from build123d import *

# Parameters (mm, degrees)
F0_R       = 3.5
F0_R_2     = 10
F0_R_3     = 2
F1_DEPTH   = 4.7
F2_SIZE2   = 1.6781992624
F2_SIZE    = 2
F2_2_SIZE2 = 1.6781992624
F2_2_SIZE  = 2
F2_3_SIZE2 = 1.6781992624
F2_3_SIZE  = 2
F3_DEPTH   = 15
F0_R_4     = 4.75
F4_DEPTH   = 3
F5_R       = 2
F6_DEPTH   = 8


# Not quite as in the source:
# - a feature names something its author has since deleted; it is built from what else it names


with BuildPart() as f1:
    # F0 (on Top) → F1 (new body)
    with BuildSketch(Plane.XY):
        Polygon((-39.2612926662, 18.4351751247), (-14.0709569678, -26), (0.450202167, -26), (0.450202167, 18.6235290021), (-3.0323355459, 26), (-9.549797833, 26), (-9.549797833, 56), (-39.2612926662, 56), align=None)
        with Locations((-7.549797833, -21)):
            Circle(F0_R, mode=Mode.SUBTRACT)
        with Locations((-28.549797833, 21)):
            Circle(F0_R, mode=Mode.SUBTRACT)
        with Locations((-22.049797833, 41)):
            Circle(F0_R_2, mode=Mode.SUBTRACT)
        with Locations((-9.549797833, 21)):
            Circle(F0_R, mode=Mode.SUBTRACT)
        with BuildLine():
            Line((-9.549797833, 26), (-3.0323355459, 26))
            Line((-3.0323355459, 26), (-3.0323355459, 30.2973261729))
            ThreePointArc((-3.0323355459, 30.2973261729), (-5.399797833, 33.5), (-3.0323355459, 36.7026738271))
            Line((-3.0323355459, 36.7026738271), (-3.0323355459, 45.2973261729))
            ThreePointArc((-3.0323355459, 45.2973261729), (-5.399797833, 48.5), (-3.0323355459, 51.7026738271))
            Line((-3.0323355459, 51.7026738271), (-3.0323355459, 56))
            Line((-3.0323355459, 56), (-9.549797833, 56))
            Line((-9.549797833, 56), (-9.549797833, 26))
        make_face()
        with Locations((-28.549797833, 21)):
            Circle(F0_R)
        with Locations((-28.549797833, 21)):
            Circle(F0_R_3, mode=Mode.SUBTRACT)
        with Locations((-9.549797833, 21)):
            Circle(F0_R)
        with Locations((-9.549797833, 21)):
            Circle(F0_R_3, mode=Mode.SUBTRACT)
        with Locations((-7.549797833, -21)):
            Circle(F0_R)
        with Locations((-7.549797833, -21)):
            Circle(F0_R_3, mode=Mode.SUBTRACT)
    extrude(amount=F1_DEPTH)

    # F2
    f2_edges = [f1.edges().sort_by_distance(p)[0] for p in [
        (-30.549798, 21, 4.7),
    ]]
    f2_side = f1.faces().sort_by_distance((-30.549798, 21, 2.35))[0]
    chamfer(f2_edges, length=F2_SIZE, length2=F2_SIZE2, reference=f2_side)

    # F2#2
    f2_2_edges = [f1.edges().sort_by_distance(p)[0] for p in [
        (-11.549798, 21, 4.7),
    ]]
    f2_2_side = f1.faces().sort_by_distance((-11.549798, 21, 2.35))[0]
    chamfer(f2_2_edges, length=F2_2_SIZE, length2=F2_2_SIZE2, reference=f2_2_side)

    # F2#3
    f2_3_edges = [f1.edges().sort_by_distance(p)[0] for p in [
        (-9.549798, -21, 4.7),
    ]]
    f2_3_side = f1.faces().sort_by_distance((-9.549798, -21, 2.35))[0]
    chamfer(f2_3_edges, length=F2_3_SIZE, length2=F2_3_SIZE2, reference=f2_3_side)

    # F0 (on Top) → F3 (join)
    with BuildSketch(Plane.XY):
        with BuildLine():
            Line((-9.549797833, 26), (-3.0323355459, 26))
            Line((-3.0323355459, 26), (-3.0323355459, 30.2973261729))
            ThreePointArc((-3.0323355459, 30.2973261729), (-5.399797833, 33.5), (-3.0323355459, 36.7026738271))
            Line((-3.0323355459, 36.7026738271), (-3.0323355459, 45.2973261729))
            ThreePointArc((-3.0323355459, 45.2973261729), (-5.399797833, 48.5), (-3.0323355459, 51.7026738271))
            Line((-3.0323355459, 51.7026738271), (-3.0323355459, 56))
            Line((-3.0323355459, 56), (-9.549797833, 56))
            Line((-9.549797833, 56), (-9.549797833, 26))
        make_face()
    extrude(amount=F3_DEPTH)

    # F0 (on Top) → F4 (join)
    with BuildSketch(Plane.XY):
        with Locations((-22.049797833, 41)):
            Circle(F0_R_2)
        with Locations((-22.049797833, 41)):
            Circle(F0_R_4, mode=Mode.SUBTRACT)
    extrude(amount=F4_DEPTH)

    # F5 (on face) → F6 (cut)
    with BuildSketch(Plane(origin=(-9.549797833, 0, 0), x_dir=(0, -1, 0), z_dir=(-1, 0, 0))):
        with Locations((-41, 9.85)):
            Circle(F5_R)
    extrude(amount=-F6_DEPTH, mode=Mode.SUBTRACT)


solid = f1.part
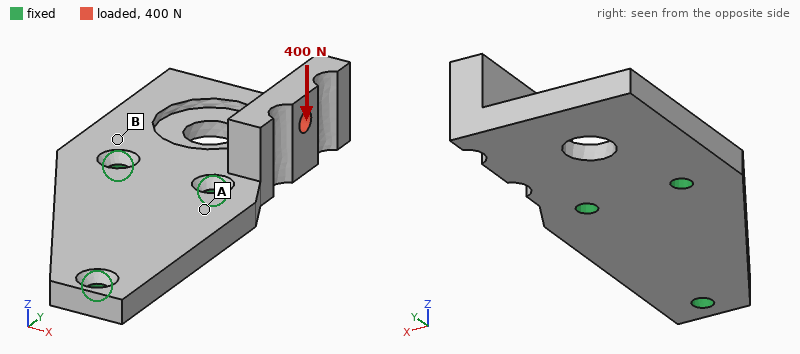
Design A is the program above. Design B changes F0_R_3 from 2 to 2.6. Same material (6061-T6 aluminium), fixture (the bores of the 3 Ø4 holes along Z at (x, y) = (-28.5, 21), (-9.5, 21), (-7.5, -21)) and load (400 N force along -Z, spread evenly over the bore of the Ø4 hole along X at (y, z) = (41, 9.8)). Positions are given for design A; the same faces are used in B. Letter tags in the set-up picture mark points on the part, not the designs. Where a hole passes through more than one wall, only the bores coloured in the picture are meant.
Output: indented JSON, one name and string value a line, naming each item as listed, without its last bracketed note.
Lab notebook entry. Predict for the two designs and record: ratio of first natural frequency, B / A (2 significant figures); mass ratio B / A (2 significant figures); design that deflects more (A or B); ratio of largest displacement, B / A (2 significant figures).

{
  "ratio of first natural frequency, B / A": "1.1",
  "mass ratio B / A": "0.99",
  "design that deflects more": "A",
  "ratio of largest displacement, B / A": "0.92"
}
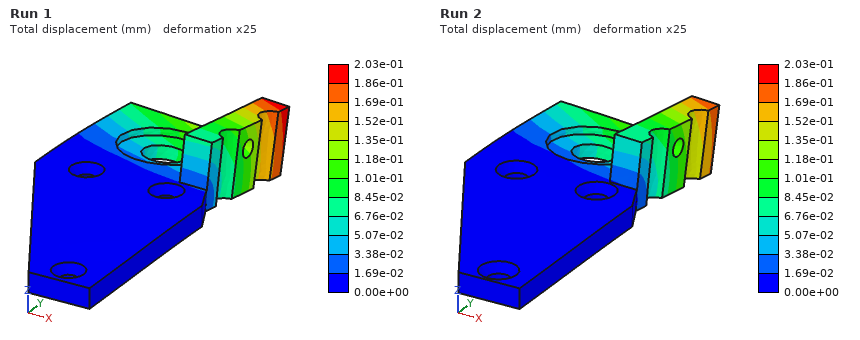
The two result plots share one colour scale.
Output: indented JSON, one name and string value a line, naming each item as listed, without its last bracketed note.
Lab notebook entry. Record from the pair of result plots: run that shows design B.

{
  "run that shows design B": "Run 2"
}
